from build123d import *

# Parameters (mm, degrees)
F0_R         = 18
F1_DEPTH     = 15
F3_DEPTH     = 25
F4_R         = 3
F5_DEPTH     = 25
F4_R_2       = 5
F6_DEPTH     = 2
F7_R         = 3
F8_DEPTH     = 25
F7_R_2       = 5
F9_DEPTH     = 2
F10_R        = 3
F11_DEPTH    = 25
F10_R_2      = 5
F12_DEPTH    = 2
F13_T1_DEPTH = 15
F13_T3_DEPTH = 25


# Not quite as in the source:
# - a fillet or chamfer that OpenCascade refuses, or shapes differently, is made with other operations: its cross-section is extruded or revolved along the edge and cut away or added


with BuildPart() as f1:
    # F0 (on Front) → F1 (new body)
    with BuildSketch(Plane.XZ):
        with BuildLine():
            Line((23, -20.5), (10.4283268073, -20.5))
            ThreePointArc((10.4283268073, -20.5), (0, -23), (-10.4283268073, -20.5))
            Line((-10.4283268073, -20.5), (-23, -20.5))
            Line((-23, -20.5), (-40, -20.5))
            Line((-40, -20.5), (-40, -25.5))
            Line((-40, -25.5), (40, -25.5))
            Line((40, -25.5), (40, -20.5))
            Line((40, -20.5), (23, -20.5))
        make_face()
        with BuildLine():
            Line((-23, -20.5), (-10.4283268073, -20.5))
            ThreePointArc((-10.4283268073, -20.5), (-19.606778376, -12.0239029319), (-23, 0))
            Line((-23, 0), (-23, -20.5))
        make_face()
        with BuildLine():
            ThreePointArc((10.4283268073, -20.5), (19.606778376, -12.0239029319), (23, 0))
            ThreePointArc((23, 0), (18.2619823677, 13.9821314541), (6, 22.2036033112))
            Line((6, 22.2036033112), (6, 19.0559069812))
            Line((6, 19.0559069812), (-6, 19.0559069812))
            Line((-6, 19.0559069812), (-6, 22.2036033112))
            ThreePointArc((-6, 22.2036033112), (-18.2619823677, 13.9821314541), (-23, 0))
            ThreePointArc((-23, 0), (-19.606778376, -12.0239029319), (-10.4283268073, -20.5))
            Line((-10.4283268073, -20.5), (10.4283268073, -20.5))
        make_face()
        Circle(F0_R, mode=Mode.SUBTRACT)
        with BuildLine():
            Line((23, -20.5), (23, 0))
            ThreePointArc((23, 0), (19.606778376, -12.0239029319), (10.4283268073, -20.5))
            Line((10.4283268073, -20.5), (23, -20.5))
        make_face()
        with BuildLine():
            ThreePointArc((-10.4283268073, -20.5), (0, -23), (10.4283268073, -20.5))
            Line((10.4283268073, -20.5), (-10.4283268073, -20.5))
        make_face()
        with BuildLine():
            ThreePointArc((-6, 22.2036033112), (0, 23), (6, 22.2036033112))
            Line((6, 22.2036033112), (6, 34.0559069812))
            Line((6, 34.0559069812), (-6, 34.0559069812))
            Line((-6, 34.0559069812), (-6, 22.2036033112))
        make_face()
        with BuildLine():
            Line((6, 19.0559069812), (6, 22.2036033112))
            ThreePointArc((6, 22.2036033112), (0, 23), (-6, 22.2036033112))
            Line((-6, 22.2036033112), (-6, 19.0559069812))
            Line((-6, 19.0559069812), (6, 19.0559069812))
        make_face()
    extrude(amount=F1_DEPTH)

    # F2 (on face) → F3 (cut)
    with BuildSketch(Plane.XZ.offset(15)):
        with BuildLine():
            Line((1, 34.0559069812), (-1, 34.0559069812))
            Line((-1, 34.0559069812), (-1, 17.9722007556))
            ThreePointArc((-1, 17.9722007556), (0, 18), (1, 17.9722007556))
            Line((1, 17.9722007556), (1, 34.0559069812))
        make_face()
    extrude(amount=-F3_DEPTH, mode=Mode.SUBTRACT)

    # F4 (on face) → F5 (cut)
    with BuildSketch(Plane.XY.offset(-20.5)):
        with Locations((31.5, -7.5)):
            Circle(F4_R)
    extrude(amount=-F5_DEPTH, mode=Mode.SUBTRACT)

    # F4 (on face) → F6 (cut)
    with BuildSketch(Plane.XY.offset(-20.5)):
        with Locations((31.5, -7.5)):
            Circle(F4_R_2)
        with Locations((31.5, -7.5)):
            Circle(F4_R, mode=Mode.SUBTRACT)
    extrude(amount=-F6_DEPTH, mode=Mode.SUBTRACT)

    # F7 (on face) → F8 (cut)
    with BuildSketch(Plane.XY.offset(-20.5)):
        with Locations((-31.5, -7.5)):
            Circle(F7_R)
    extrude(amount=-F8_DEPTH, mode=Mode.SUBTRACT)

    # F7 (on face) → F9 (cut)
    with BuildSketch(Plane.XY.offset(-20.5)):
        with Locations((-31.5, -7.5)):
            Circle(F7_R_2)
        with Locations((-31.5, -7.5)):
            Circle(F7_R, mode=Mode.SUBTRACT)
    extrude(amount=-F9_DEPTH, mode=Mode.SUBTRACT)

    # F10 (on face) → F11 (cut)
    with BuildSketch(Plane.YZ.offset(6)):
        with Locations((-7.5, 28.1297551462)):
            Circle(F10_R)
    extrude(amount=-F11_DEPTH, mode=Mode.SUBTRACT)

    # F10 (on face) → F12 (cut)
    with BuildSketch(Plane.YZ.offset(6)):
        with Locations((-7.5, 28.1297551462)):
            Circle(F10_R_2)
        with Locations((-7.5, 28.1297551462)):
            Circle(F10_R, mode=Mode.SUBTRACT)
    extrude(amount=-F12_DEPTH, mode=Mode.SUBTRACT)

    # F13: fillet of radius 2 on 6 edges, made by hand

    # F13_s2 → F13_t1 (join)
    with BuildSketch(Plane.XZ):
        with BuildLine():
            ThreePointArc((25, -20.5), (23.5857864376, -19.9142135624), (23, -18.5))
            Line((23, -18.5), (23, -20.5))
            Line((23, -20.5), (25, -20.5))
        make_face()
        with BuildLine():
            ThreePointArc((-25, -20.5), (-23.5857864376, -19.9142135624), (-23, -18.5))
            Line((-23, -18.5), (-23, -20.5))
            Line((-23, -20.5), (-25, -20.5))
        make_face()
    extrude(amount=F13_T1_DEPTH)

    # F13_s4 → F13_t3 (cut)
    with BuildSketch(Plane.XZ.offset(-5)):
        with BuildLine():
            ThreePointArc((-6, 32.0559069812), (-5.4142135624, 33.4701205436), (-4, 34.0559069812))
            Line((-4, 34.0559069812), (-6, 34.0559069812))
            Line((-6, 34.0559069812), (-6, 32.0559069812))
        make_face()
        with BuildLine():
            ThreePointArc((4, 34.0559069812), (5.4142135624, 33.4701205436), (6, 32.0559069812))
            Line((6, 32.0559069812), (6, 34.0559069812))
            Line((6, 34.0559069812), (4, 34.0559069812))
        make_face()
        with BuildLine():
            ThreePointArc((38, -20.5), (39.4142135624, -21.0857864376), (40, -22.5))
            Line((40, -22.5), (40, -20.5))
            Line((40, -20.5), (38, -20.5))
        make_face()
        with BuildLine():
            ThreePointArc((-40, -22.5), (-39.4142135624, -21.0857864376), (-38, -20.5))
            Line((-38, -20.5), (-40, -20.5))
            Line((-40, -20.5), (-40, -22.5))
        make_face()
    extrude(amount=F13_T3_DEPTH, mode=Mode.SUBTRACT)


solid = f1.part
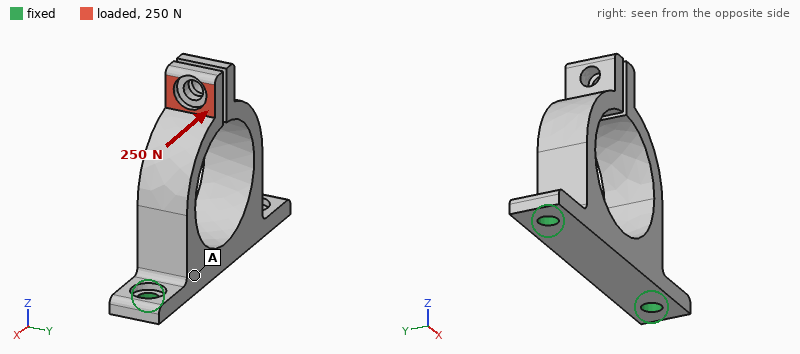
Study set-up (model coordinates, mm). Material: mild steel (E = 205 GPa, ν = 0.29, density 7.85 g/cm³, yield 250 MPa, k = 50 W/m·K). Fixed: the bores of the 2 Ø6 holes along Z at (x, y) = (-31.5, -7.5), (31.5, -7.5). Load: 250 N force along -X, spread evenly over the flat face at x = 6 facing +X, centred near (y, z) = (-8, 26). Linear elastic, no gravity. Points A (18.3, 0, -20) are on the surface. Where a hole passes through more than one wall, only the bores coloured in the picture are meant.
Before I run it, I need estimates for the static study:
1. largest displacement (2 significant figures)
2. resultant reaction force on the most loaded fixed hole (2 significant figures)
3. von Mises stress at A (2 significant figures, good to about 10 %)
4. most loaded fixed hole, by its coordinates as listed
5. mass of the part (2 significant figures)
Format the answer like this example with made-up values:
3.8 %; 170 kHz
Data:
0.21 mm; 590 N; 21 MPa; (-31.5, -7.5); 140 g
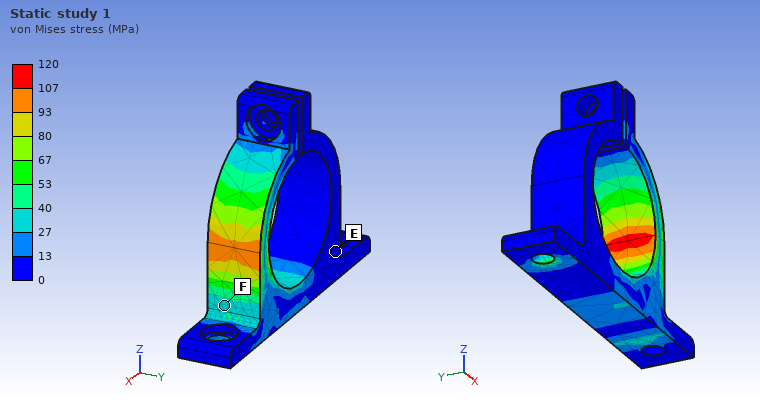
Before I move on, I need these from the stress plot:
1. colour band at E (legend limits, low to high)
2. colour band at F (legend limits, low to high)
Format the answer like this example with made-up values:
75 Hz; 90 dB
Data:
0 to 13 MPa; 27 to 40 MPa
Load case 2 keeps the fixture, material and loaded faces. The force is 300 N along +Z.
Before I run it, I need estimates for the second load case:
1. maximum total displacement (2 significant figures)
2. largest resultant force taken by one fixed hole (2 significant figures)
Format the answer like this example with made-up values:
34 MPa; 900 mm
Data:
0.12 mm; 350 N
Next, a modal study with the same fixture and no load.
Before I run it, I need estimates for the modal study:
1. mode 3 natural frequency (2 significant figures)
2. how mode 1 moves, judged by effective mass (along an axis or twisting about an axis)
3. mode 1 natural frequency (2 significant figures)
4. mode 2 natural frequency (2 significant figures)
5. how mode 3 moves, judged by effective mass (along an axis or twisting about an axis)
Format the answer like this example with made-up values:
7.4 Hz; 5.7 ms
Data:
1800 Hz; along Y; 1400 Hz; 1600 Hz; along X
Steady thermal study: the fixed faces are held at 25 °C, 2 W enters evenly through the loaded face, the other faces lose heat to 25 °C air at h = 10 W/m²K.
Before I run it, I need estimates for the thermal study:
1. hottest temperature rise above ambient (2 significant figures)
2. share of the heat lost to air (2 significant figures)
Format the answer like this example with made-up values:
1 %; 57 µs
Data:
27 K; 24 %
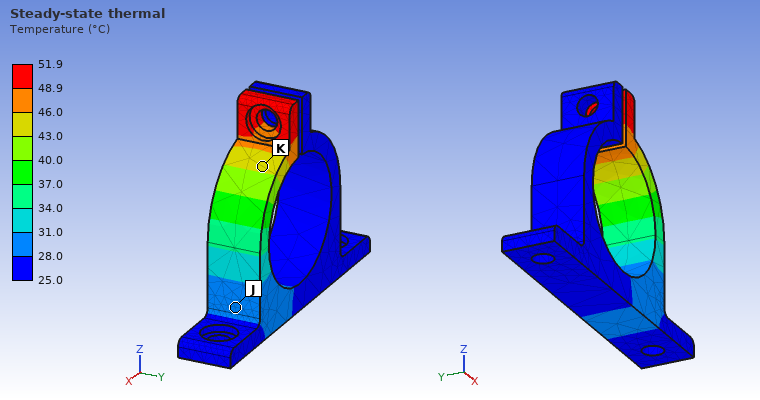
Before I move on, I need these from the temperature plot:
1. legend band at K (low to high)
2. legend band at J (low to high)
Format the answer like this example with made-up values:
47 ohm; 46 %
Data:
43.0 to 46.0 °C; 28.0 to 31.0 °C
